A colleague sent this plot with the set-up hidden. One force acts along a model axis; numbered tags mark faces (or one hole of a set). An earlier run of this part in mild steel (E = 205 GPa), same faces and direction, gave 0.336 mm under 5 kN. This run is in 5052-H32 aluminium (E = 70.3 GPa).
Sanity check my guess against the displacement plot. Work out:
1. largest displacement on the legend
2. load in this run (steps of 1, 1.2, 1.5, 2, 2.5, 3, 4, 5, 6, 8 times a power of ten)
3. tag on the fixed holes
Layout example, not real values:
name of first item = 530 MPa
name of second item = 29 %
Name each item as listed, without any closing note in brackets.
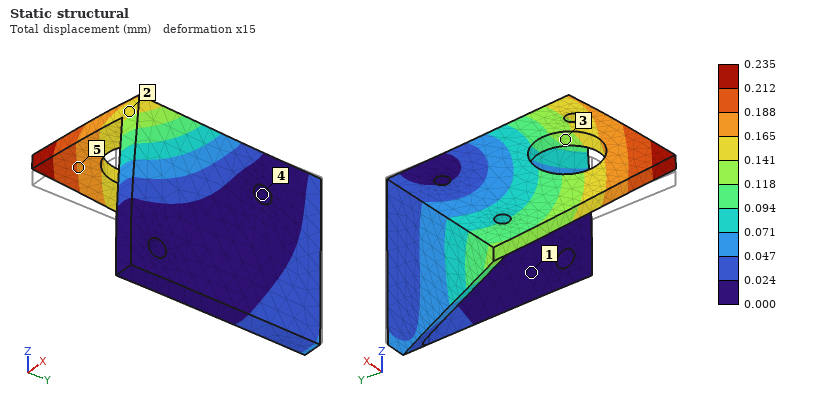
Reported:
largest displacement on the legend = 0.235 mm
load in this run = 1.2 kN
tag on the fixed holes = 4
